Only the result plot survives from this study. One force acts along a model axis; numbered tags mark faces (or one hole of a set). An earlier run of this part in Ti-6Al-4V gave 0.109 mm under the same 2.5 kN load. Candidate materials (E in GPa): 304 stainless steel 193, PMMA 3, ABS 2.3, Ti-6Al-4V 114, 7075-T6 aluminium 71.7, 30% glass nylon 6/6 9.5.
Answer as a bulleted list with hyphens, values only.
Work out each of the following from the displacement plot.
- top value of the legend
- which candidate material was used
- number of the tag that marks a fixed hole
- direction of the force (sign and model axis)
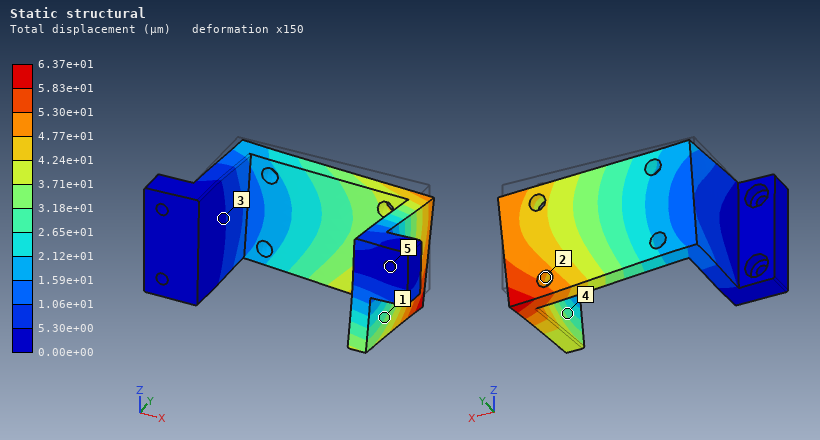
- 6.37e+01 µm
- 304 stainless steel
- 5
- -Z
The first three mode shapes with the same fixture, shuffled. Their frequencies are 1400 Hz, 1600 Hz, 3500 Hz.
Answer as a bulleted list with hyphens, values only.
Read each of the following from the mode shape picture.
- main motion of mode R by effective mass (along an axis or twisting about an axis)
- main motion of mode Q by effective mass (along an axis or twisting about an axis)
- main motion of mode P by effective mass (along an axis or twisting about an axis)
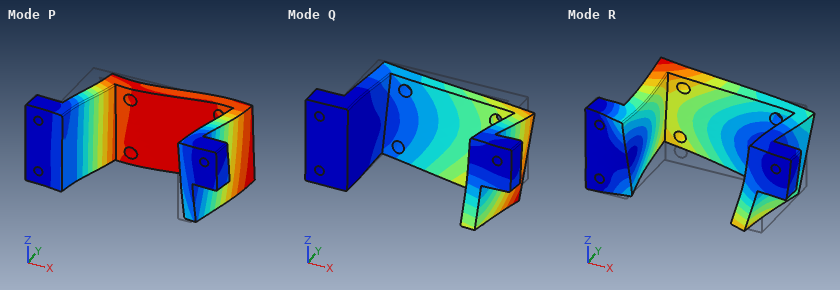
- along Z
- along Z
- along X
